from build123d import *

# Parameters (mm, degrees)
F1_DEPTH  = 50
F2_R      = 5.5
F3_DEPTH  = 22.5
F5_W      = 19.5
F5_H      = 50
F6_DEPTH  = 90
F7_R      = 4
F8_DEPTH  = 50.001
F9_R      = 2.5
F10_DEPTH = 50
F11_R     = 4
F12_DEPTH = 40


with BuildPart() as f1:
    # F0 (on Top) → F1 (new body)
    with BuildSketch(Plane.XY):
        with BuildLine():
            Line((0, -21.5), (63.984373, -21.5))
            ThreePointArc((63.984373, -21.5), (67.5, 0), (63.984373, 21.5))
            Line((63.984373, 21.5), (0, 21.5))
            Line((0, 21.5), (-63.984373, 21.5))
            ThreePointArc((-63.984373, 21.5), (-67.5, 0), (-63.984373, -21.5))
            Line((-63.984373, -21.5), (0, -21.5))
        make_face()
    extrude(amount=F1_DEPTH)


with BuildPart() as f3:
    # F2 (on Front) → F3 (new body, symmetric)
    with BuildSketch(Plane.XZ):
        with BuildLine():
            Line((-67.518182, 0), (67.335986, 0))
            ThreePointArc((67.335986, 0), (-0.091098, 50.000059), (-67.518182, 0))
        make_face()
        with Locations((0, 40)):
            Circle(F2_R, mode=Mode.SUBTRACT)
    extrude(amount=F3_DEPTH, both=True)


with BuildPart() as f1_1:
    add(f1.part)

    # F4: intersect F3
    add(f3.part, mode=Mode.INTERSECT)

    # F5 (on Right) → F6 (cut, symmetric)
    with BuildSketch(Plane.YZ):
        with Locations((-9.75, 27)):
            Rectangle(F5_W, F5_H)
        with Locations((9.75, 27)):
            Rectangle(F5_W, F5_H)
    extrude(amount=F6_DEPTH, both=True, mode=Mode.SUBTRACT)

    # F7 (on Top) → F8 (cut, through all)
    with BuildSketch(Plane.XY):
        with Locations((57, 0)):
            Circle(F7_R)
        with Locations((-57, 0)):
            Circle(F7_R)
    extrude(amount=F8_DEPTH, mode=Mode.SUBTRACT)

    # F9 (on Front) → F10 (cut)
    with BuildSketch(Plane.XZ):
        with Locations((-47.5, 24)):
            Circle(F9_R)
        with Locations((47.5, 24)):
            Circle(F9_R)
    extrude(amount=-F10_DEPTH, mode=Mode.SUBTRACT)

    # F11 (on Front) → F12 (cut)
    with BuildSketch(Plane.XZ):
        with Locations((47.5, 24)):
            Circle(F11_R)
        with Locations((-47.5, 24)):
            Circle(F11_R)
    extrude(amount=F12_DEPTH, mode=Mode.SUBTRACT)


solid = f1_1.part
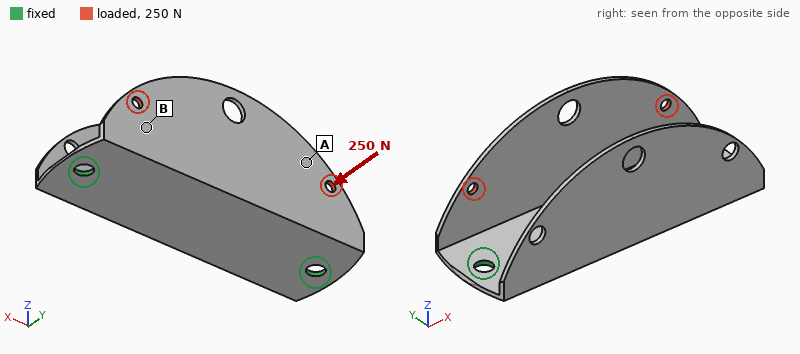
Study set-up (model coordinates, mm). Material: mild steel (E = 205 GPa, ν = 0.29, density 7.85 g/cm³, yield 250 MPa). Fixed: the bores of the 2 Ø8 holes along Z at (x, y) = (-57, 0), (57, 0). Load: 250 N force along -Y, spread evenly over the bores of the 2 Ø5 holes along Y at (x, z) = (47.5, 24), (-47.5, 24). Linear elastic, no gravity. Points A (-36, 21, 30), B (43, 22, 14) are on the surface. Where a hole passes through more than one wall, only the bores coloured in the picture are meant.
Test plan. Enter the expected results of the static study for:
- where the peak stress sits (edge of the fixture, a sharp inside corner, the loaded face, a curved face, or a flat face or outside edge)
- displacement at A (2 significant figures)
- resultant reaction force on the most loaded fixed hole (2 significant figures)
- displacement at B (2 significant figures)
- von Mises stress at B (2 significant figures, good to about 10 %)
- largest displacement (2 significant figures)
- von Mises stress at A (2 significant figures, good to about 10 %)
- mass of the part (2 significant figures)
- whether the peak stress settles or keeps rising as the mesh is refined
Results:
edge of the fixture
0.28 mm
130 N
0.15 mm
42 MPa
0.40 mm
17 MPa
230 g
keeps rising
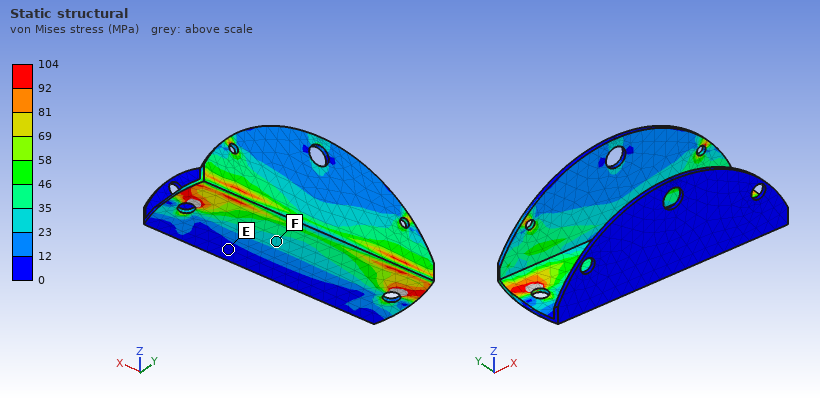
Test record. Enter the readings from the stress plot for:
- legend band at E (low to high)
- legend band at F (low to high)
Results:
0 to 12 MPa
23 to 35 MPa
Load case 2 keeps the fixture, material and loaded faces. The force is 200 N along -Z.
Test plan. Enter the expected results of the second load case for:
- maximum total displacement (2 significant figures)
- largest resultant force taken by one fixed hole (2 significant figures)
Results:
0.12 mm
100 N
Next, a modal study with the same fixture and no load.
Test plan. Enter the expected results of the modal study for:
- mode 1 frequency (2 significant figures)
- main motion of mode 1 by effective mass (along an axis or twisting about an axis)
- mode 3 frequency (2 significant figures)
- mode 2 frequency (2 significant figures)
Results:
530 Hz
along Y
1200 Hz
600 Hz
